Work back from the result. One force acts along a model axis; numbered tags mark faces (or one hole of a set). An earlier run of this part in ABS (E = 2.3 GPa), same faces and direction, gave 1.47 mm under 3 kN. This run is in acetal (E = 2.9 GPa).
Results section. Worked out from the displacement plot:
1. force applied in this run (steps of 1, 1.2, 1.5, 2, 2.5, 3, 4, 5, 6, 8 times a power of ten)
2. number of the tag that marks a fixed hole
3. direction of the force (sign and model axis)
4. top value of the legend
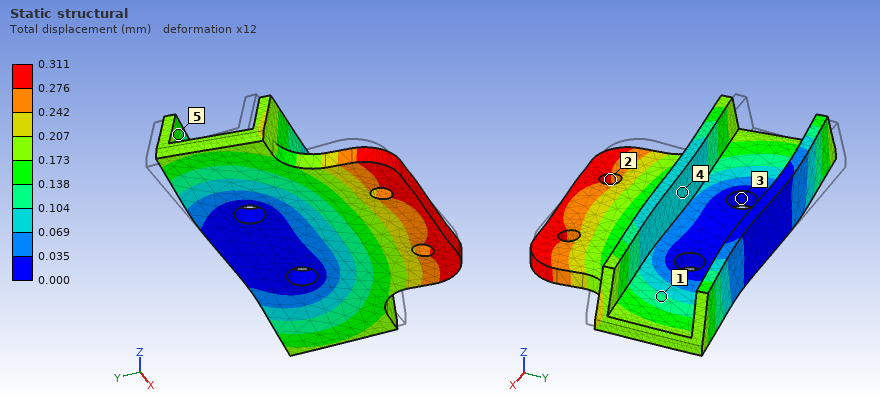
800 N
3
+X
0.311 mm
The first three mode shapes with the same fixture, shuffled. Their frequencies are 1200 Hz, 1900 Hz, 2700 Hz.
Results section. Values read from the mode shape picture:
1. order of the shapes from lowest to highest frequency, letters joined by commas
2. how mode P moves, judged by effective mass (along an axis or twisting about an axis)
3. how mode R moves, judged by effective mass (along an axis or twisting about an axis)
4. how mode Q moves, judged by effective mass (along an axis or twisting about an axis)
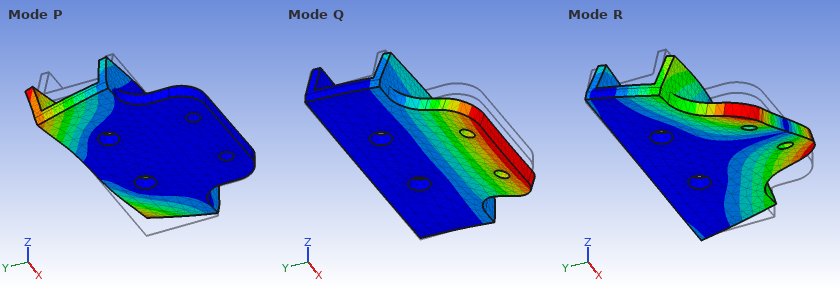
Q, R, P
twisting about Y
twisting about Y
along Z
